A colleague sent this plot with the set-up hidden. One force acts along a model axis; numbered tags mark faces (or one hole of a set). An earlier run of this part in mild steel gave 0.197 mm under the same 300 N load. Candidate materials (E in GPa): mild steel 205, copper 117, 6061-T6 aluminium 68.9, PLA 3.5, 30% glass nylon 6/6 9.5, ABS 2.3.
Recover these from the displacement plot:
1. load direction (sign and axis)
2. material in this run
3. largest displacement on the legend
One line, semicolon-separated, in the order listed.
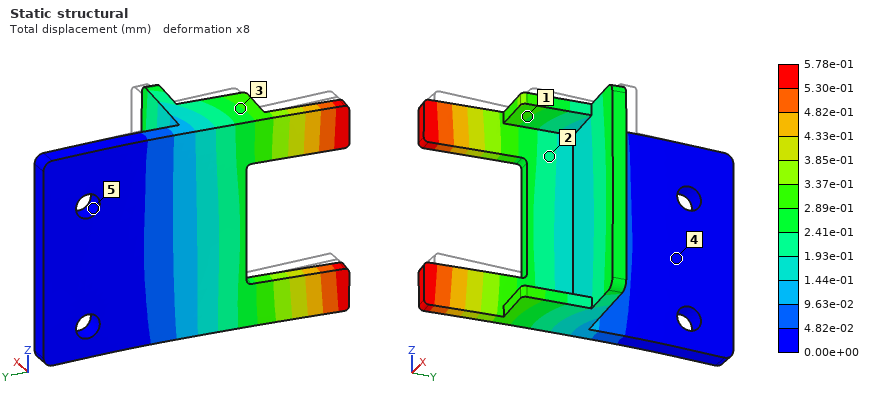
-X; 6061-T6 aluminium; 5.78e-01 mm
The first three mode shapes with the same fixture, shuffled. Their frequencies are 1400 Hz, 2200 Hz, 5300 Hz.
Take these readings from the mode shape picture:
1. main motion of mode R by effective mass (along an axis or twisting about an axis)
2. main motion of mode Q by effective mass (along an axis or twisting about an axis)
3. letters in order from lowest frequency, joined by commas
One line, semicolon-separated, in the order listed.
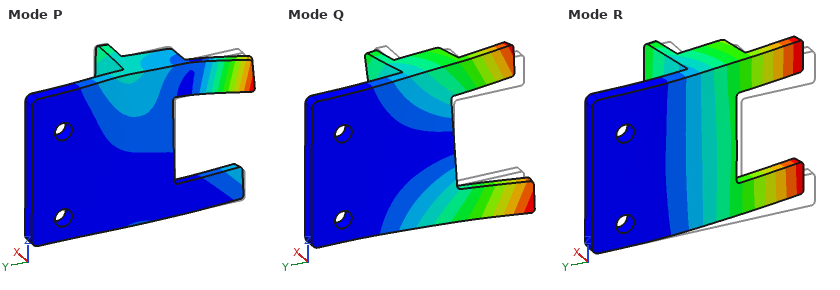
along X; twisting about Y; R, Q, P
